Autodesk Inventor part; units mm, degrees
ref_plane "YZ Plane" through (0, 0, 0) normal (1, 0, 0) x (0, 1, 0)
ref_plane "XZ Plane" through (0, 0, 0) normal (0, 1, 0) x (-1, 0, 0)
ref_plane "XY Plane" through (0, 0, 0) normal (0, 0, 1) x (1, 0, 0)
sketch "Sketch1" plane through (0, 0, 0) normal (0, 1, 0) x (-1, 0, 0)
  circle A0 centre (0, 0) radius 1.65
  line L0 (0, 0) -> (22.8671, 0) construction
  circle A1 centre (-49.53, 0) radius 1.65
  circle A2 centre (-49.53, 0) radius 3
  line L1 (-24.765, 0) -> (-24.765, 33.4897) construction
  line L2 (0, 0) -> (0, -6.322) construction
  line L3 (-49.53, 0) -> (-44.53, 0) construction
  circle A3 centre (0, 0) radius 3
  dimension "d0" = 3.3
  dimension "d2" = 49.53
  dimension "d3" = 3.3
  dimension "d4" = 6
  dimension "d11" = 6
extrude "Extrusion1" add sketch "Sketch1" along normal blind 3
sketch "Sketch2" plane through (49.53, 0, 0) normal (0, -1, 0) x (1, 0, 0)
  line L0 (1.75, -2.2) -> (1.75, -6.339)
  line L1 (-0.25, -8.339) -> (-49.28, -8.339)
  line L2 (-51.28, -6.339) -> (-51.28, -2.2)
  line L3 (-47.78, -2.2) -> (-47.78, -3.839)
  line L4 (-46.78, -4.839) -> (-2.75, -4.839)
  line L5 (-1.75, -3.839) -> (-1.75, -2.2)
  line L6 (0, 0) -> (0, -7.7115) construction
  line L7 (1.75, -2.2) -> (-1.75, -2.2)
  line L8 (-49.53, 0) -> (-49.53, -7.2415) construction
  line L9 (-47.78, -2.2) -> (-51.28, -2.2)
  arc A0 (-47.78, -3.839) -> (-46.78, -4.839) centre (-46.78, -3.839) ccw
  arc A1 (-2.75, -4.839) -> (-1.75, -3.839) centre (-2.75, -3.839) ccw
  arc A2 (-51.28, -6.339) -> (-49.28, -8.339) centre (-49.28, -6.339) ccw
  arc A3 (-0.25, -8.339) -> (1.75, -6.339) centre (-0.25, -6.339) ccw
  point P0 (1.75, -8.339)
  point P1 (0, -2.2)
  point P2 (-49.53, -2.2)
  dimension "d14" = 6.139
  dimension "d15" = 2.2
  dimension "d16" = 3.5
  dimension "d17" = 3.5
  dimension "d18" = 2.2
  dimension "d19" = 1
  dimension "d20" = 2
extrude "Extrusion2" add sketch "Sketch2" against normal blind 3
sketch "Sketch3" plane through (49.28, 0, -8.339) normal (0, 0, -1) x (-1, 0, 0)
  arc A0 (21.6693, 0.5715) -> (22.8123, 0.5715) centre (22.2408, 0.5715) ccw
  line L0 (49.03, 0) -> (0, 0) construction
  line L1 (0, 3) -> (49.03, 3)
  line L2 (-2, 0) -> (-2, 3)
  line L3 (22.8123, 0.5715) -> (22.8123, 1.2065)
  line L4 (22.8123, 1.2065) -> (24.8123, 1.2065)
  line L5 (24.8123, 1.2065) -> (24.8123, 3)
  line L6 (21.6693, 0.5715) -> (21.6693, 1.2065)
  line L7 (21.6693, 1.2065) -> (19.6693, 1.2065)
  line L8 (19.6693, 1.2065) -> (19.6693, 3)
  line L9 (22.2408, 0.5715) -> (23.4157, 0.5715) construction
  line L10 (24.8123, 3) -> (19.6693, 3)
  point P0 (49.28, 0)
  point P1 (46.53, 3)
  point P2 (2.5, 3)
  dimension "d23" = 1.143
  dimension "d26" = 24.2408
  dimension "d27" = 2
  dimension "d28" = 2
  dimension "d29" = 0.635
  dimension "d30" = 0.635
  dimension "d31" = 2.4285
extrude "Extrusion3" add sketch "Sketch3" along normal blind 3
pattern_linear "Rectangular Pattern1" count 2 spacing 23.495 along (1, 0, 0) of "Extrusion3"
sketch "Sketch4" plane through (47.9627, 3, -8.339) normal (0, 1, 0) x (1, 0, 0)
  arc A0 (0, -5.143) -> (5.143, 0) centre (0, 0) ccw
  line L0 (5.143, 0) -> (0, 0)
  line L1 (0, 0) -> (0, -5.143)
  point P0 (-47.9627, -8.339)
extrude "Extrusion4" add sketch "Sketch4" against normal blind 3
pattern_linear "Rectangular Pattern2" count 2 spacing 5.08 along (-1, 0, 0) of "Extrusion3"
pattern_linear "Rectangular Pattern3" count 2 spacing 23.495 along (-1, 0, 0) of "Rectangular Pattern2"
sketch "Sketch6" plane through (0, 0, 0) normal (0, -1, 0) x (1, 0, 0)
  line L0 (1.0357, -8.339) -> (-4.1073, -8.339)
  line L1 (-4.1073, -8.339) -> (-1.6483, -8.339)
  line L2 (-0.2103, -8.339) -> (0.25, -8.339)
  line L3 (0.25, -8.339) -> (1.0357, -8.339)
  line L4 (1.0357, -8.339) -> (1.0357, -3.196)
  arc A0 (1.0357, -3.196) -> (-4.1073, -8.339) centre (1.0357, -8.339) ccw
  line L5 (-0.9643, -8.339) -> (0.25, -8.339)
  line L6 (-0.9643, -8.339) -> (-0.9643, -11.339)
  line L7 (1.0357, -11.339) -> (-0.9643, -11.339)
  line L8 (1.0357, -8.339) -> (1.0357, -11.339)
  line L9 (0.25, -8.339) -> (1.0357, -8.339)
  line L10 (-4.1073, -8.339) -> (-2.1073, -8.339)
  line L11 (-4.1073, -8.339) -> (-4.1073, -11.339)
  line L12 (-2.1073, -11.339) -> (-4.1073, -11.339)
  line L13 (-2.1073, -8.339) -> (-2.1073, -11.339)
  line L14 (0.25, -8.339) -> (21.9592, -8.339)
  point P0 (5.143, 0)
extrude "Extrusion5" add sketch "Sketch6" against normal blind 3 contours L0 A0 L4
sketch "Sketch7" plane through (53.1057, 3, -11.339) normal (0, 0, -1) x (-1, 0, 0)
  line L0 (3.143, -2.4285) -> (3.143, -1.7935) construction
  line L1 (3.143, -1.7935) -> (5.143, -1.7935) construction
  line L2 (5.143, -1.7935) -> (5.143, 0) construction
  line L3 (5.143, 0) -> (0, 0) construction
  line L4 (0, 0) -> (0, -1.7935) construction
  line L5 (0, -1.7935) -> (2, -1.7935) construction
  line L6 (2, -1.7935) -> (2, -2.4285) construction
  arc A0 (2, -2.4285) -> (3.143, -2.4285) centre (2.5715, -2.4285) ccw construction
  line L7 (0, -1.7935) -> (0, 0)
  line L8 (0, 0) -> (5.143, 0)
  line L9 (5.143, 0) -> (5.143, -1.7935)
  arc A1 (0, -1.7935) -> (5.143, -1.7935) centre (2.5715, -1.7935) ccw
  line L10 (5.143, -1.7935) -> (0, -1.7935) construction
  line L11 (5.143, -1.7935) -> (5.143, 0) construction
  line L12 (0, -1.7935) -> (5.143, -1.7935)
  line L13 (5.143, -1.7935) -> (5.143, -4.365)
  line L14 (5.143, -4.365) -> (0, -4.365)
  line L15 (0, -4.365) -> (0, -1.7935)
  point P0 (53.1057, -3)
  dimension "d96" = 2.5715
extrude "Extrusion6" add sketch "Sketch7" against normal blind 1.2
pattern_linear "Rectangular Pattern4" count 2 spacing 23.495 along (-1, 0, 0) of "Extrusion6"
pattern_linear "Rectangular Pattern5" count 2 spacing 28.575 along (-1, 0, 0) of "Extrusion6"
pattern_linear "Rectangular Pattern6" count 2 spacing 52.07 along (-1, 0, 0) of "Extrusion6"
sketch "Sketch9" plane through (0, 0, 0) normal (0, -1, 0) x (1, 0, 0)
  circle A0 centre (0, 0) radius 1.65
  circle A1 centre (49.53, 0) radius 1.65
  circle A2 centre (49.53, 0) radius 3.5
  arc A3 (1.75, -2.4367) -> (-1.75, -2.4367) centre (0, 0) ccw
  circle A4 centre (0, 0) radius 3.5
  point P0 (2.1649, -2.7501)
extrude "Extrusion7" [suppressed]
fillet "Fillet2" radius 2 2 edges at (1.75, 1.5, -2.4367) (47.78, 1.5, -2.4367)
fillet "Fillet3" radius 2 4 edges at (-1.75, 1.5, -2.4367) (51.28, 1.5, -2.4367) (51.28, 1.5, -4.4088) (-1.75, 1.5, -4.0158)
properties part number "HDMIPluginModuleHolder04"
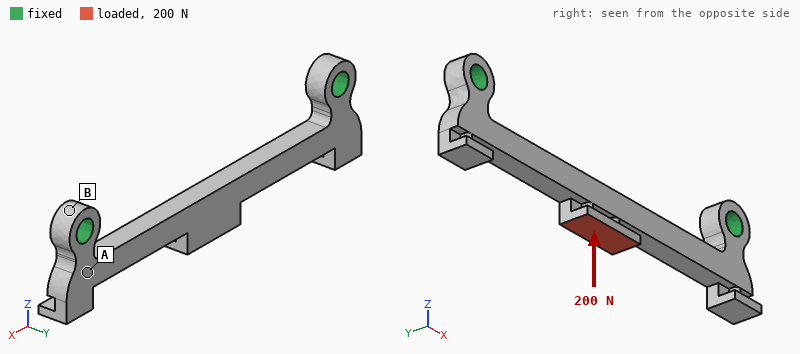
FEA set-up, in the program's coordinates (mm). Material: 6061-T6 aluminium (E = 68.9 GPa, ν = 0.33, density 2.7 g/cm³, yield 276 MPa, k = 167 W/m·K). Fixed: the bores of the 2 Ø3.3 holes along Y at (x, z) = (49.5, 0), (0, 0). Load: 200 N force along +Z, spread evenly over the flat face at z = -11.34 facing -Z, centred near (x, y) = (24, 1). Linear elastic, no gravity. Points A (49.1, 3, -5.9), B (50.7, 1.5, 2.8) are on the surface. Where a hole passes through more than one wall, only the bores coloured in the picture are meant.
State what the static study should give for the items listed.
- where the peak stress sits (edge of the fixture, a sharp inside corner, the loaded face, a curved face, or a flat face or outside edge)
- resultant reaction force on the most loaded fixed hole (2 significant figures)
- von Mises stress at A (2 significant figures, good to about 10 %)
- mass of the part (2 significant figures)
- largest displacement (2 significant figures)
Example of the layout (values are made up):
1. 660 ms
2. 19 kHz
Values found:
1. a curved face
2. 210 N
3. 58 MPa
4. 2.5 g
5. 0.15 mm
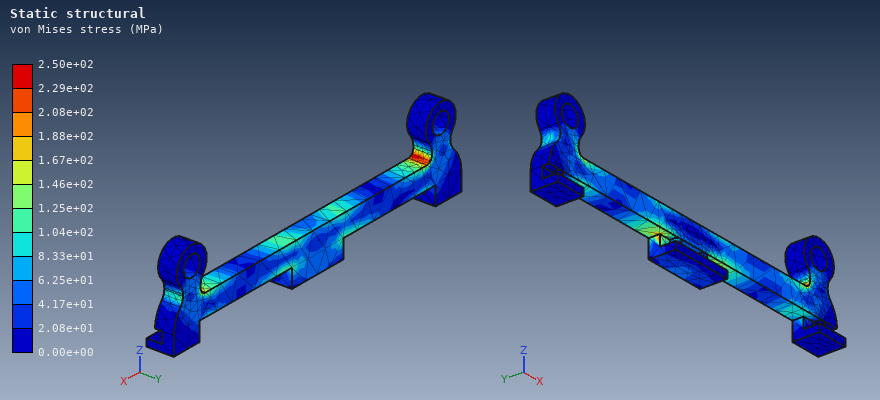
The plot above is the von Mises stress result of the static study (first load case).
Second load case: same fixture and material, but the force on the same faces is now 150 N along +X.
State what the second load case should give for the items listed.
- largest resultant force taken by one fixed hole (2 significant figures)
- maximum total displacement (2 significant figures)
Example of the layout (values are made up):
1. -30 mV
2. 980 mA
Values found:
1. 79 N
2. 19 µm
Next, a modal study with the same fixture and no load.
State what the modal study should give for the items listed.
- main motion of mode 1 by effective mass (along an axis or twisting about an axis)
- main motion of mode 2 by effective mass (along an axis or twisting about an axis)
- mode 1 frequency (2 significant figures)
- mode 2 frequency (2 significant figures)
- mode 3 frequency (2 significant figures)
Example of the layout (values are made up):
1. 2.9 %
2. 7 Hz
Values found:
1. along Y
2. along Z
3. 4300 Hz
4. 6500 Hz
5. 13 kHz
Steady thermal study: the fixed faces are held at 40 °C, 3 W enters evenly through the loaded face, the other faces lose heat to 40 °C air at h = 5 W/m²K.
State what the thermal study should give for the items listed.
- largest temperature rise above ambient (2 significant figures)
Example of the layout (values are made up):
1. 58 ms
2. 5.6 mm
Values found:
1. 24 K
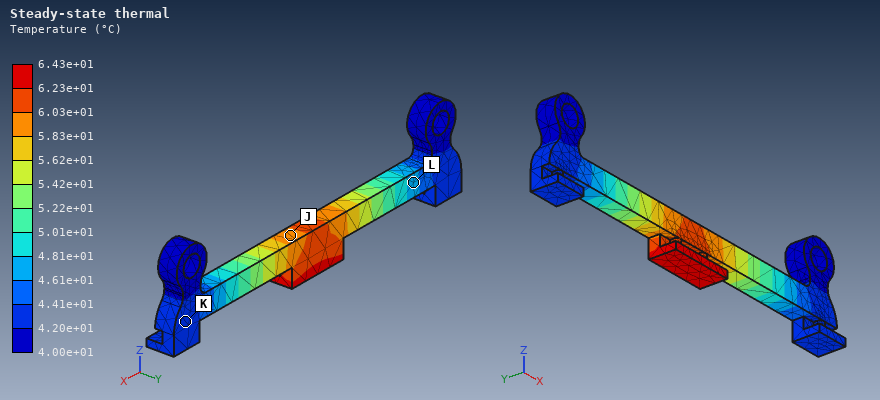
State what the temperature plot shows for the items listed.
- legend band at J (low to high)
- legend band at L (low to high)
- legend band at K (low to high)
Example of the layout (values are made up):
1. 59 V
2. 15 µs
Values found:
1. 5.83e+01 to 6.03e+01 °C
2. 4.61e+01 to 4.81e+01 °C
3. 4.20e+01 to 4.41e+01 °C
